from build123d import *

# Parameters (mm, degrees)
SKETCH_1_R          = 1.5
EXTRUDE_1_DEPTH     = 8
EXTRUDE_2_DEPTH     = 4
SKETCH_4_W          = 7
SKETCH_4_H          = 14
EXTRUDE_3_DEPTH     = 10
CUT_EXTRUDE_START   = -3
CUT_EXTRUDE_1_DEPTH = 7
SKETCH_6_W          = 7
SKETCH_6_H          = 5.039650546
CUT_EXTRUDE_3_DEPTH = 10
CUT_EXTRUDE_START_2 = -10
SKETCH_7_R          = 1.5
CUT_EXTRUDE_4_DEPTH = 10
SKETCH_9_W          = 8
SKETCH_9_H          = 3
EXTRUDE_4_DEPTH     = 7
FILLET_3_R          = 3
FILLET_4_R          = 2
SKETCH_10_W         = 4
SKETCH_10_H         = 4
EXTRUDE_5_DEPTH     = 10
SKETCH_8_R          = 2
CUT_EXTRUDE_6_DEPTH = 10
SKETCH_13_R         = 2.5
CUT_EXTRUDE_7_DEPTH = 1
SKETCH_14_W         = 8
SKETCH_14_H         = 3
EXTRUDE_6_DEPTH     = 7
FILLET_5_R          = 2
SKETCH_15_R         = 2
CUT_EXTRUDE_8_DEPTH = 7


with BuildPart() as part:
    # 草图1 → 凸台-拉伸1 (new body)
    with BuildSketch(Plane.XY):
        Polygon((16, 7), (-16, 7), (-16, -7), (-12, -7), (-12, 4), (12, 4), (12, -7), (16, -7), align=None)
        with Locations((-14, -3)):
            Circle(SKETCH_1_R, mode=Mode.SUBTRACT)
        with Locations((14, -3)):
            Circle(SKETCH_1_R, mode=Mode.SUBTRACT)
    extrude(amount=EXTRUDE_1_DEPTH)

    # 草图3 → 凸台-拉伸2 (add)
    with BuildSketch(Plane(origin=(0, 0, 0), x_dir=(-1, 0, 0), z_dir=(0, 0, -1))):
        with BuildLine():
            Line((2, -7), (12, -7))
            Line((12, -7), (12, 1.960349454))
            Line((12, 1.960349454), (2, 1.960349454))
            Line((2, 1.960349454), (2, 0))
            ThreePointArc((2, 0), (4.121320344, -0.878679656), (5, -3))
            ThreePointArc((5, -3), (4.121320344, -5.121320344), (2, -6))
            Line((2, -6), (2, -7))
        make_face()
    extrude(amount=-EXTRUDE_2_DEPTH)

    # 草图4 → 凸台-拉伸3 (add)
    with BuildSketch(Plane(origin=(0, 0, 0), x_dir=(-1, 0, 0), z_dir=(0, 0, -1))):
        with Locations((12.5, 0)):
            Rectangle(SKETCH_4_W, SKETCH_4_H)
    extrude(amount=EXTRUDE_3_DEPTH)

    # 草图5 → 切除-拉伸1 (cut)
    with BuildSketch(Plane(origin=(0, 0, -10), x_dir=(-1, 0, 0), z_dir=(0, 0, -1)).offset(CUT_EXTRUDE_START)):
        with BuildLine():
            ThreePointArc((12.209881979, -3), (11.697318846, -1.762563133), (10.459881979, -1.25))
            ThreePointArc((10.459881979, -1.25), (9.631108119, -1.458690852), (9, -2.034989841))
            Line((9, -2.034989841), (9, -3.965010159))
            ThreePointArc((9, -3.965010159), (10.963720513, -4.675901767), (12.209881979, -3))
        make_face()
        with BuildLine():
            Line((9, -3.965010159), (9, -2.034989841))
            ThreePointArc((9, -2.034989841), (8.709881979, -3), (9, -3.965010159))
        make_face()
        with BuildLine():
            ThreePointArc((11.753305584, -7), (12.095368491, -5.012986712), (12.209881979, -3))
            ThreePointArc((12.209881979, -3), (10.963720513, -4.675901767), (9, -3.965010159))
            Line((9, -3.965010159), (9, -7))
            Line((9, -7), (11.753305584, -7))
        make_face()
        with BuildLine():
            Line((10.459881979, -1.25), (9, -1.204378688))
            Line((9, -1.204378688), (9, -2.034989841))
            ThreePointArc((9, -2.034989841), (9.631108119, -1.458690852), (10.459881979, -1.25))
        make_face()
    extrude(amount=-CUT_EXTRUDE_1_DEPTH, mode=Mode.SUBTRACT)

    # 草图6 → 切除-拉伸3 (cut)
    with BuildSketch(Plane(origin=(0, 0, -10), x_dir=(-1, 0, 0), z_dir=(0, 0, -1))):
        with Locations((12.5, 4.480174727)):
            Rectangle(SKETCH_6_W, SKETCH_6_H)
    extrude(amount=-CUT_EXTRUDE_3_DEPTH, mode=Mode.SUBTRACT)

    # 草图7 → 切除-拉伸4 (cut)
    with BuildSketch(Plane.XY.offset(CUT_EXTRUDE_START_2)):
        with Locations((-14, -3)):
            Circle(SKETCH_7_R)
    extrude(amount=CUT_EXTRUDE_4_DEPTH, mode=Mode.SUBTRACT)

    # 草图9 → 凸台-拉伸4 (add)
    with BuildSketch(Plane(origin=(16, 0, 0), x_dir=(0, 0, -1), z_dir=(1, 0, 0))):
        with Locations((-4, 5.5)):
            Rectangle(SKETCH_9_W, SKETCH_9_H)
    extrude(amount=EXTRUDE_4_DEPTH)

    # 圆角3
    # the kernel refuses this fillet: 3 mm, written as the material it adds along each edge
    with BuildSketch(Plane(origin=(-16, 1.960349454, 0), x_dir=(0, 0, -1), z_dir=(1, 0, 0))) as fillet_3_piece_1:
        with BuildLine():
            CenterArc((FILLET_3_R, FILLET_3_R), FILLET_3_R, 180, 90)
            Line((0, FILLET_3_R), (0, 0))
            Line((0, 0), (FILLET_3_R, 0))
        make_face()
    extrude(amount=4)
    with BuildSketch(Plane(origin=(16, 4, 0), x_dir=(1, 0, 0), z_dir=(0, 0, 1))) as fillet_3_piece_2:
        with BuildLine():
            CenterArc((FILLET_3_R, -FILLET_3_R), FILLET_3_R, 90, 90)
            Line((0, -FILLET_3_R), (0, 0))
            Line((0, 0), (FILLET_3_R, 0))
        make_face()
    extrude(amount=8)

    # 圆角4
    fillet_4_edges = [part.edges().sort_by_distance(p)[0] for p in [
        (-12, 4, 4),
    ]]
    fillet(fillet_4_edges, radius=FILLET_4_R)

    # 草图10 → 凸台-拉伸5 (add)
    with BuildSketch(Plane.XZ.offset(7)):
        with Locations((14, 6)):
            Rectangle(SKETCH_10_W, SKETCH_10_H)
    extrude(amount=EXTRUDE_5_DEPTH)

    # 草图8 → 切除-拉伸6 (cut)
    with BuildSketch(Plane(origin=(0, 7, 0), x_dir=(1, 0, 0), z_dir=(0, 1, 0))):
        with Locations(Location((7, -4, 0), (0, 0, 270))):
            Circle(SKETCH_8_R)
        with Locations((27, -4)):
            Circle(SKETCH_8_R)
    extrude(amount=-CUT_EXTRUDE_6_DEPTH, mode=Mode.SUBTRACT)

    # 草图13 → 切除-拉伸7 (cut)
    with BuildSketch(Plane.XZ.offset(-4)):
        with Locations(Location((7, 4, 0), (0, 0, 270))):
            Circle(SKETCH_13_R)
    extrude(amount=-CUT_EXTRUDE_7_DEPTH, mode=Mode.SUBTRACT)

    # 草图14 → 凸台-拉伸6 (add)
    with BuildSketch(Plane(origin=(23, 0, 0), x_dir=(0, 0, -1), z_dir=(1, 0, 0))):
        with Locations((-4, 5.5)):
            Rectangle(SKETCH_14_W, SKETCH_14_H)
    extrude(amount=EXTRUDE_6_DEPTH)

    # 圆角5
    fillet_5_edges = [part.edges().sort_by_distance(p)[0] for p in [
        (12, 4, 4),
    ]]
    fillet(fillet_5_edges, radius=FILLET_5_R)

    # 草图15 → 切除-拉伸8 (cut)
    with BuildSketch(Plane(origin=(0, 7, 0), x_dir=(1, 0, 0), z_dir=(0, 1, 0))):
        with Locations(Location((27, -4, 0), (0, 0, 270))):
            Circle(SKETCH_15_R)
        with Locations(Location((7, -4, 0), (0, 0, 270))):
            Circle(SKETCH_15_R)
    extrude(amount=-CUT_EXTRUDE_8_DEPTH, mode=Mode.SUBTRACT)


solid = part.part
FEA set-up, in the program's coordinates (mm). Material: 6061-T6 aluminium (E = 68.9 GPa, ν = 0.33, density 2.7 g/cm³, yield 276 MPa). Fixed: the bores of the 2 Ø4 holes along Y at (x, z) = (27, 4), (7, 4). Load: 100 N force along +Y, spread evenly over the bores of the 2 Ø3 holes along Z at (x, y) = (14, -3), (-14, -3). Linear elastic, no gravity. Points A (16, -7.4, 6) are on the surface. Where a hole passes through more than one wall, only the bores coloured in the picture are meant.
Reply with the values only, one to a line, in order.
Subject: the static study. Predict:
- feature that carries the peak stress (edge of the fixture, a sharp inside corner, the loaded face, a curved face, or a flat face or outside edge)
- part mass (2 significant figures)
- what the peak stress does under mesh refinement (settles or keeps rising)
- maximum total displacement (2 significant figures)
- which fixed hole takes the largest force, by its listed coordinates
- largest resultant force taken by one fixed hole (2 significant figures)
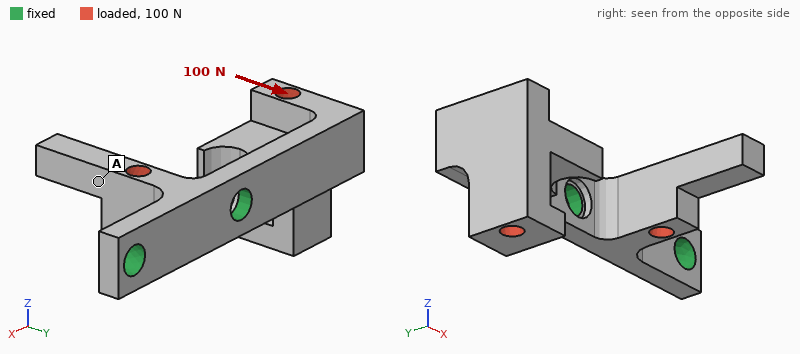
edge of the fixture
6.9 g
keeps rising
0.31 mm
(7, 4)
97 N
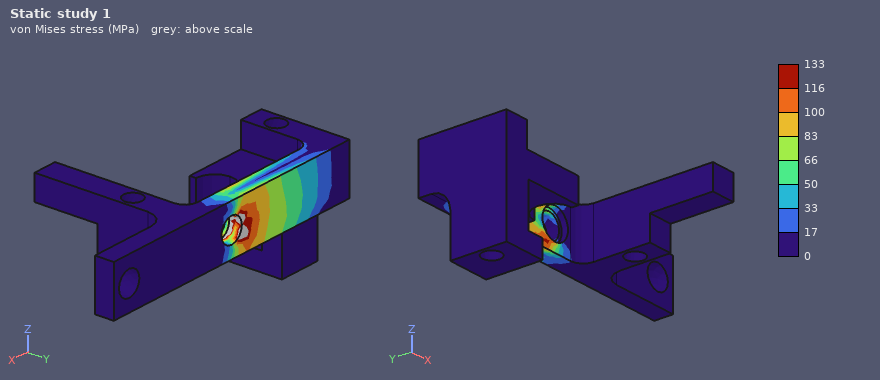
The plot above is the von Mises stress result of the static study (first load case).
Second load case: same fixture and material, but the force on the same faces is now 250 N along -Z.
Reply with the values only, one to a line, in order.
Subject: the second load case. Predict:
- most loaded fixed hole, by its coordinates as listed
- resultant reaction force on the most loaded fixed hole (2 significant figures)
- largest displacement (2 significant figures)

(7, 4)
270 N
0.40 mm
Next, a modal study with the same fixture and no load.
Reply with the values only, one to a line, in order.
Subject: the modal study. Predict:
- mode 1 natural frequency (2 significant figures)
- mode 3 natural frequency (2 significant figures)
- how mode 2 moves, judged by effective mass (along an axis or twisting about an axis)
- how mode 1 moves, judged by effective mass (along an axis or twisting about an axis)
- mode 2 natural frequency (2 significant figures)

1600 Hz
5500 Hz
along Z
along Y
2500 Hz
